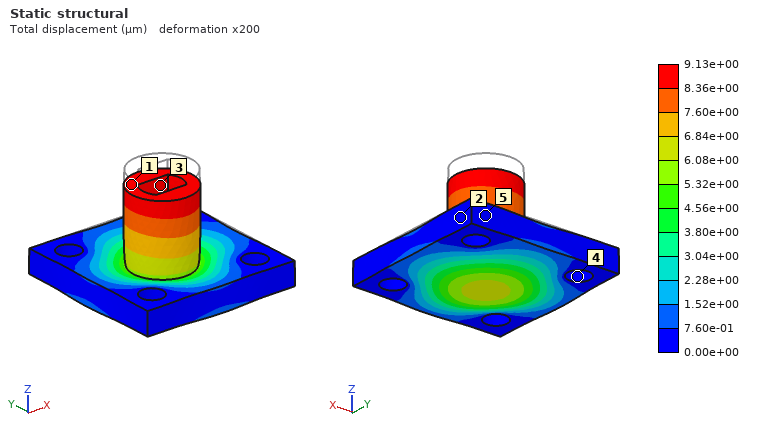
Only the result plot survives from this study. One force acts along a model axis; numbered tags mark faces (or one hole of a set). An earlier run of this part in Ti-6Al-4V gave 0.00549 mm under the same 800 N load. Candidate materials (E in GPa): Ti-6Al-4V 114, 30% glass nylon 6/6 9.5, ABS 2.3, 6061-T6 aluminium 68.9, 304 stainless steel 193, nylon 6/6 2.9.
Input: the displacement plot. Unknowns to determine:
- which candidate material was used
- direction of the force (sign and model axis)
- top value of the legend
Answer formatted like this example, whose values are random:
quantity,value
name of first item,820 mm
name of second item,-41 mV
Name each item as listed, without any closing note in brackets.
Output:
quantity,value
which candidate material was used,6061-T6 aluminium
direction of the force,-Z
top value of the legend,9.13e+00 µm
